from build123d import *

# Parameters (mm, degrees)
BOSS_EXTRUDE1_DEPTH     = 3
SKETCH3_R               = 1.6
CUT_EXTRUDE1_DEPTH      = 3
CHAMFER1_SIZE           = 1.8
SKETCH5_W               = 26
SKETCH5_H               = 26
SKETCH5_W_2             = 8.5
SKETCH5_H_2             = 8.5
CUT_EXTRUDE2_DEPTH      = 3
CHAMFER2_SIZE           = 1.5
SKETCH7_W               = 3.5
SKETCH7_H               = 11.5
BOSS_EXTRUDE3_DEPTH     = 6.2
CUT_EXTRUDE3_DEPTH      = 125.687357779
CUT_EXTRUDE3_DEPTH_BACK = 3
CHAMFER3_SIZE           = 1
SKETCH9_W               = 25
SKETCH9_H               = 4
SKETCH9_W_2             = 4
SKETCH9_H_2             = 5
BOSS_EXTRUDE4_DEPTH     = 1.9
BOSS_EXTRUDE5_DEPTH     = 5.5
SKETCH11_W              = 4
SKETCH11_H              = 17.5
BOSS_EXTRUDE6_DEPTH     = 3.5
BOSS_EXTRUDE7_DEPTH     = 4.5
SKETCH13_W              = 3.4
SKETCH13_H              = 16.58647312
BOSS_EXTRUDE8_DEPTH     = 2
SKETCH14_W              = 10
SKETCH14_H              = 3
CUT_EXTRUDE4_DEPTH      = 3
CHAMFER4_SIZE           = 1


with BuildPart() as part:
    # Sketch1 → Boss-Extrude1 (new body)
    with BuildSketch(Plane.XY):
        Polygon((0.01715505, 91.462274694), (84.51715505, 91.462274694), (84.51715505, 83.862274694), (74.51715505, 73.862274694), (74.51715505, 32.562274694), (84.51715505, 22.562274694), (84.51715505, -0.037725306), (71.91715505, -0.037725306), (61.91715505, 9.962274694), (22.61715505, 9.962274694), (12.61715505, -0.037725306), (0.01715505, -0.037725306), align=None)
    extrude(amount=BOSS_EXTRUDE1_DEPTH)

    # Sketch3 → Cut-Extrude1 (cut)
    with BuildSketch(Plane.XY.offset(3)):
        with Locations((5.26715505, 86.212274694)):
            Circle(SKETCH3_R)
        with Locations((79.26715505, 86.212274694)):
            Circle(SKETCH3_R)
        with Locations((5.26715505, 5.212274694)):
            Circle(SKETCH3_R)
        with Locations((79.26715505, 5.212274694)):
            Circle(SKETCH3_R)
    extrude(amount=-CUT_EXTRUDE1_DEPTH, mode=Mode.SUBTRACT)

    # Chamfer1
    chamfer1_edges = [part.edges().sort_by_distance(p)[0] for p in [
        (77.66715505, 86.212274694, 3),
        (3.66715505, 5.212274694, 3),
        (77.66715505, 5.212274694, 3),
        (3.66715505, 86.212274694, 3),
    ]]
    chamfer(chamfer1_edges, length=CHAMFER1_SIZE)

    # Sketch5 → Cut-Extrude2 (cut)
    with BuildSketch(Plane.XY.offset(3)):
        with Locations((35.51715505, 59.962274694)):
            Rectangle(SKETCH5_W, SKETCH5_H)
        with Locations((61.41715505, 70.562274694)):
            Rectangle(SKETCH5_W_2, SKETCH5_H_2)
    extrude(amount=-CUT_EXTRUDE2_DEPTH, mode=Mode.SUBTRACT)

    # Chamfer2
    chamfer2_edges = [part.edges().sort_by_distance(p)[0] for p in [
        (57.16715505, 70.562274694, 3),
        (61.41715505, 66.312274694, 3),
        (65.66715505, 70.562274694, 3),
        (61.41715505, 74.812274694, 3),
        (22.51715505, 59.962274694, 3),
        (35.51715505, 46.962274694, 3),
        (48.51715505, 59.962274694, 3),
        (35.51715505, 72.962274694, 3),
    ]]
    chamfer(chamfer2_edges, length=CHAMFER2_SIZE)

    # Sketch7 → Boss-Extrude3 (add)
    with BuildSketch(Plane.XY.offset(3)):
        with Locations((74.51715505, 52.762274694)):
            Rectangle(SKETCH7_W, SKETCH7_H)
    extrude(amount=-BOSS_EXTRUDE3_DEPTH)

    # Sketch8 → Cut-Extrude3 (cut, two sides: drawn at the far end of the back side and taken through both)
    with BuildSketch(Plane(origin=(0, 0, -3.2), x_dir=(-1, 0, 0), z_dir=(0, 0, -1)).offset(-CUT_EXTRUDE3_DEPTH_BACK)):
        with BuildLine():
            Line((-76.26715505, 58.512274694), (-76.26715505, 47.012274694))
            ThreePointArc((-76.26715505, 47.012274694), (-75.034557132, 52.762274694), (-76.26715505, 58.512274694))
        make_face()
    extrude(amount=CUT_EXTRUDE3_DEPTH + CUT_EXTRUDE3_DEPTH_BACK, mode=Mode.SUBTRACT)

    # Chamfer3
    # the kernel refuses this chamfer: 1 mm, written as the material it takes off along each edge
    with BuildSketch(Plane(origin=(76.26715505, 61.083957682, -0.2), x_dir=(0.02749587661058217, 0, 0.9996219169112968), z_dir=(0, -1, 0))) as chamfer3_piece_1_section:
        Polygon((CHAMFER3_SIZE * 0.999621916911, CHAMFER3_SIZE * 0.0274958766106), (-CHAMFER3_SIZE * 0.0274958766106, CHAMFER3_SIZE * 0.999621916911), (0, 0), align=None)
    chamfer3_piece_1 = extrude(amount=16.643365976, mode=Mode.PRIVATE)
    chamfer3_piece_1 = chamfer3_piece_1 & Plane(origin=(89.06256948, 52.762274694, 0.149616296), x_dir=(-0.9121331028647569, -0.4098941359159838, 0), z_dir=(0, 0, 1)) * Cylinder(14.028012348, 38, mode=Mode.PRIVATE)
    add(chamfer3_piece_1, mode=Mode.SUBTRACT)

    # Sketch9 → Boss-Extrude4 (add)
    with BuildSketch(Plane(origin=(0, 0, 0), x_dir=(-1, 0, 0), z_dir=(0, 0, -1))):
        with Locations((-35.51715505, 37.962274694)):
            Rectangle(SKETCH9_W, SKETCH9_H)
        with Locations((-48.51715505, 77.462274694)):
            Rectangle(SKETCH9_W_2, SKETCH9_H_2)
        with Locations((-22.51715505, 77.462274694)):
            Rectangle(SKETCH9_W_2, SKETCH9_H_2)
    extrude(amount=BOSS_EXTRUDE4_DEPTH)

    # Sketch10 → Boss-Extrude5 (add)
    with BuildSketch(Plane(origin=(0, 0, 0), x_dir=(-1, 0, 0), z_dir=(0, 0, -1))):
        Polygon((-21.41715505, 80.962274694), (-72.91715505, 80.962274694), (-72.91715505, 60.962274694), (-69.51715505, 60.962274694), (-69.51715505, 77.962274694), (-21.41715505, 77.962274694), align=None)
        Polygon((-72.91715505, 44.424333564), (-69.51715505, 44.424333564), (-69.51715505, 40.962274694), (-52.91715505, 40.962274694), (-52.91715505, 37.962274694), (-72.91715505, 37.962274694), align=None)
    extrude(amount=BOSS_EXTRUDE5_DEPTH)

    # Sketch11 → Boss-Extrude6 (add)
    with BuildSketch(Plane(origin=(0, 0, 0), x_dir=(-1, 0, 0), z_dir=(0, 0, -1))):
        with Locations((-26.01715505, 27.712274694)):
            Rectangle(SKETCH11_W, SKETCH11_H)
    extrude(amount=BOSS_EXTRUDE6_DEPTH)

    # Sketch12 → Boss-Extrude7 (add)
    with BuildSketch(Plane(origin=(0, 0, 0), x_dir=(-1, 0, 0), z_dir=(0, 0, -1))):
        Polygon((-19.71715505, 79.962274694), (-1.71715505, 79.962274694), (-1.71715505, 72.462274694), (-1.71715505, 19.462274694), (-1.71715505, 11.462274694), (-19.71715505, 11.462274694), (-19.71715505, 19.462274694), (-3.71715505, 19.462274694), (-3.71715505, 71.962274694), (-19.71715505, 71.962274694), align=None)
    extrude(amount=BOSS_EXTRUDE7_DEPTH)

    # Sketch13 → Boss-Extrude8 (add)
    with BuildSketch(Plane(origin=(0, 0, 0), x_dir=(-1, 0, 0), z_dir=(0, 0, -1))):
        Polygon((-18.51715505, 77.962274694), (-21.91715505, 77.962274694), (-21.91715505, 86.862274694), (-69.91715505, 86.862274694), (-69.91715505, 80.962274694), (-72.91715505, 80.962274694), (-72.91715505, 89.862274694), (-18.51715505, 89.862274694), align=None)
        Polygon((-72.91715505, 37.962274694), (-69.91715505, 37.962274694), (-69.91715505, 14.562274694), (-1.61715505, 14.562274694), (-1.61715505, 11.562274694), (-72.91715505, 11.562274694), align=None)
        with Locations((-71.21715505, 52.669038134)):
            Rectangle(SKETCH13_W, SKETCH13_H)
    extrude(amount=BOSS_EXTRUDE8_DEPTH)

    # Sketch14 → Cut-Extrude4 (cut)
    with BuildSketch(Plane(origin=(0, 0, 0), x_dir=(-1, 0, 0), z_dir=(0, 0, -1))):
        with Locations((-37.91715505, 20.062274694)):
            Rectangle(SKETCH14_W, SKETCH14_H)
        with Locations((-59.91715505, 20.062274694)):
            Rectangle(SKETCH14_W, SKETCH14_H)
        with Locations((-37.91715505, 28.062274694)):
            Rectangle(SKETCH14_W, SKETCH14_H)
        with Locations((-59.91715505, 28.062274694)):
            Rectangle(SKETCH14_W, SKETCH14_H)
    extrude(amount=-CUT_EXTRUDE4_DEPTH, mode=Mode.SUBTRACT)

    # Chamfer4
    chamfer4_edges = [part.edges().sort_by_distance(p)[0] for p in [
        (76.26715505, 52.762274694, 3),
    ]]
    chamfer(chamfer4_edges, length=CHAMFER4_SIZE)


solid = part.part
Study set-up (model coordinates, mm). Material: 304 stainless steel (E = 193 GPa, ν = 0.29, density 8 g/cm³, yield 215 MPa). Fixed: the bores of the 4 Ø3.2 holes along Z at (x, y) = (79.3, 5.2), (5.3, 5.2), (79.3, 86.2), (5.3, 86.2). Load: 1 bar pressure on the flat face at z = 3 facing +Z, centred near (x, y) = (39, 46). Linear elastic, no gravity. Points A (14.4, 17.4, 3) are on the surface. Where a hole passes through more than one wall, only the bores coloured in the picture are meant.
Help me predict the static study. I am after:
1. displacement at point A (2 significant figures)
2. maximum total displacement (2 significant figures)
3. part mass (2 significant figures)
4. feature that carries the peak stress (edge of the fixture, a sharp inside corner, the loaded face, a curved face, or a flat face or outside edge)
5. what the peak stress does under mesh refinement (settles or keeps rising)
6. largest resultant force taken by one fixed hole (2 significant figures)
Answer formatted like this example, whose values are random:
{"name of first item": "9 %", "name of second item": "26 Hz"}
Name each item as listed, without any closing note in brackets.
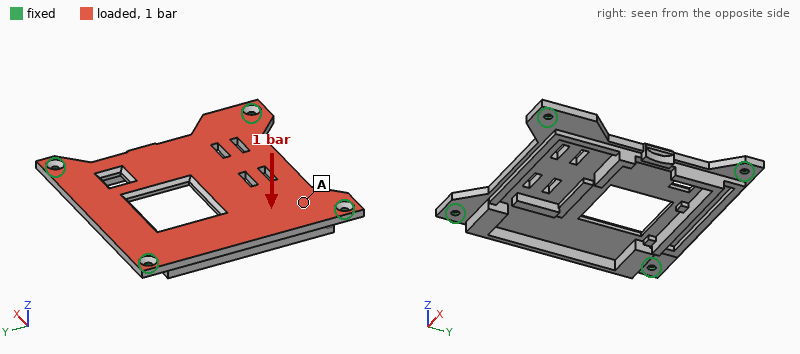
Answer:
{"displacement at point A": "20 µm", "maximum total displacement": "56 µm", "part mass": "180 g", "feature that carries the peak stress": "edge of the fixture", "what the peak stress does under mesh refinement": "keeps rising", "largest resultant force taken by one fixed hole": "160 N"}
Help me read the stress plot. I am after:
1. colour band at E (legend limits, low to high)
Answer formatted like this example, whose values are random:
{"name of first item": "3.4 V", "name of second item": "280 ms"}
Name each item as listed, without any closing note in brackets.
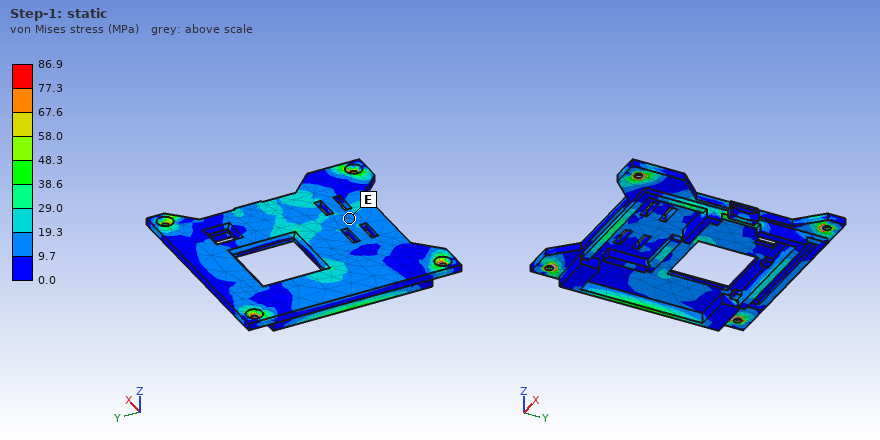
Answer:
{"colour band at E": "9.7 to 19.3 MPa"}
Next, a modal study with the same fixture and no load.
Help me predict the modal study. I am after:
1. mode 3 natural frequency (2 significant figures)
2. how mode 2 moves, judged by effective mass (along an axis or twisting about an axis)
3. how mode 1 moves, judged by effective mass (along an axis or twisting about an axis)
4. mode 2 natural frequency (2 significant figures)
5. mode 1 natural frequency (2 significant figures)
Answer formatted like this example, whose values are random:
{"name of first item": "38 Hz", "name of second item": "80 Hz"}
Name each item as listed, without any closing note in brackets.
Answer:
{"mode 3 natural frequency": "3200 Hz", "how mode 2 moves, judged by effective mass": "twisting about Y", "how mode 1 moves, judged by effective mass": "along Z", "mode 2 natural frequency": "2700 Hz", "mode 1 natural frequency": "1500 Hz"}
